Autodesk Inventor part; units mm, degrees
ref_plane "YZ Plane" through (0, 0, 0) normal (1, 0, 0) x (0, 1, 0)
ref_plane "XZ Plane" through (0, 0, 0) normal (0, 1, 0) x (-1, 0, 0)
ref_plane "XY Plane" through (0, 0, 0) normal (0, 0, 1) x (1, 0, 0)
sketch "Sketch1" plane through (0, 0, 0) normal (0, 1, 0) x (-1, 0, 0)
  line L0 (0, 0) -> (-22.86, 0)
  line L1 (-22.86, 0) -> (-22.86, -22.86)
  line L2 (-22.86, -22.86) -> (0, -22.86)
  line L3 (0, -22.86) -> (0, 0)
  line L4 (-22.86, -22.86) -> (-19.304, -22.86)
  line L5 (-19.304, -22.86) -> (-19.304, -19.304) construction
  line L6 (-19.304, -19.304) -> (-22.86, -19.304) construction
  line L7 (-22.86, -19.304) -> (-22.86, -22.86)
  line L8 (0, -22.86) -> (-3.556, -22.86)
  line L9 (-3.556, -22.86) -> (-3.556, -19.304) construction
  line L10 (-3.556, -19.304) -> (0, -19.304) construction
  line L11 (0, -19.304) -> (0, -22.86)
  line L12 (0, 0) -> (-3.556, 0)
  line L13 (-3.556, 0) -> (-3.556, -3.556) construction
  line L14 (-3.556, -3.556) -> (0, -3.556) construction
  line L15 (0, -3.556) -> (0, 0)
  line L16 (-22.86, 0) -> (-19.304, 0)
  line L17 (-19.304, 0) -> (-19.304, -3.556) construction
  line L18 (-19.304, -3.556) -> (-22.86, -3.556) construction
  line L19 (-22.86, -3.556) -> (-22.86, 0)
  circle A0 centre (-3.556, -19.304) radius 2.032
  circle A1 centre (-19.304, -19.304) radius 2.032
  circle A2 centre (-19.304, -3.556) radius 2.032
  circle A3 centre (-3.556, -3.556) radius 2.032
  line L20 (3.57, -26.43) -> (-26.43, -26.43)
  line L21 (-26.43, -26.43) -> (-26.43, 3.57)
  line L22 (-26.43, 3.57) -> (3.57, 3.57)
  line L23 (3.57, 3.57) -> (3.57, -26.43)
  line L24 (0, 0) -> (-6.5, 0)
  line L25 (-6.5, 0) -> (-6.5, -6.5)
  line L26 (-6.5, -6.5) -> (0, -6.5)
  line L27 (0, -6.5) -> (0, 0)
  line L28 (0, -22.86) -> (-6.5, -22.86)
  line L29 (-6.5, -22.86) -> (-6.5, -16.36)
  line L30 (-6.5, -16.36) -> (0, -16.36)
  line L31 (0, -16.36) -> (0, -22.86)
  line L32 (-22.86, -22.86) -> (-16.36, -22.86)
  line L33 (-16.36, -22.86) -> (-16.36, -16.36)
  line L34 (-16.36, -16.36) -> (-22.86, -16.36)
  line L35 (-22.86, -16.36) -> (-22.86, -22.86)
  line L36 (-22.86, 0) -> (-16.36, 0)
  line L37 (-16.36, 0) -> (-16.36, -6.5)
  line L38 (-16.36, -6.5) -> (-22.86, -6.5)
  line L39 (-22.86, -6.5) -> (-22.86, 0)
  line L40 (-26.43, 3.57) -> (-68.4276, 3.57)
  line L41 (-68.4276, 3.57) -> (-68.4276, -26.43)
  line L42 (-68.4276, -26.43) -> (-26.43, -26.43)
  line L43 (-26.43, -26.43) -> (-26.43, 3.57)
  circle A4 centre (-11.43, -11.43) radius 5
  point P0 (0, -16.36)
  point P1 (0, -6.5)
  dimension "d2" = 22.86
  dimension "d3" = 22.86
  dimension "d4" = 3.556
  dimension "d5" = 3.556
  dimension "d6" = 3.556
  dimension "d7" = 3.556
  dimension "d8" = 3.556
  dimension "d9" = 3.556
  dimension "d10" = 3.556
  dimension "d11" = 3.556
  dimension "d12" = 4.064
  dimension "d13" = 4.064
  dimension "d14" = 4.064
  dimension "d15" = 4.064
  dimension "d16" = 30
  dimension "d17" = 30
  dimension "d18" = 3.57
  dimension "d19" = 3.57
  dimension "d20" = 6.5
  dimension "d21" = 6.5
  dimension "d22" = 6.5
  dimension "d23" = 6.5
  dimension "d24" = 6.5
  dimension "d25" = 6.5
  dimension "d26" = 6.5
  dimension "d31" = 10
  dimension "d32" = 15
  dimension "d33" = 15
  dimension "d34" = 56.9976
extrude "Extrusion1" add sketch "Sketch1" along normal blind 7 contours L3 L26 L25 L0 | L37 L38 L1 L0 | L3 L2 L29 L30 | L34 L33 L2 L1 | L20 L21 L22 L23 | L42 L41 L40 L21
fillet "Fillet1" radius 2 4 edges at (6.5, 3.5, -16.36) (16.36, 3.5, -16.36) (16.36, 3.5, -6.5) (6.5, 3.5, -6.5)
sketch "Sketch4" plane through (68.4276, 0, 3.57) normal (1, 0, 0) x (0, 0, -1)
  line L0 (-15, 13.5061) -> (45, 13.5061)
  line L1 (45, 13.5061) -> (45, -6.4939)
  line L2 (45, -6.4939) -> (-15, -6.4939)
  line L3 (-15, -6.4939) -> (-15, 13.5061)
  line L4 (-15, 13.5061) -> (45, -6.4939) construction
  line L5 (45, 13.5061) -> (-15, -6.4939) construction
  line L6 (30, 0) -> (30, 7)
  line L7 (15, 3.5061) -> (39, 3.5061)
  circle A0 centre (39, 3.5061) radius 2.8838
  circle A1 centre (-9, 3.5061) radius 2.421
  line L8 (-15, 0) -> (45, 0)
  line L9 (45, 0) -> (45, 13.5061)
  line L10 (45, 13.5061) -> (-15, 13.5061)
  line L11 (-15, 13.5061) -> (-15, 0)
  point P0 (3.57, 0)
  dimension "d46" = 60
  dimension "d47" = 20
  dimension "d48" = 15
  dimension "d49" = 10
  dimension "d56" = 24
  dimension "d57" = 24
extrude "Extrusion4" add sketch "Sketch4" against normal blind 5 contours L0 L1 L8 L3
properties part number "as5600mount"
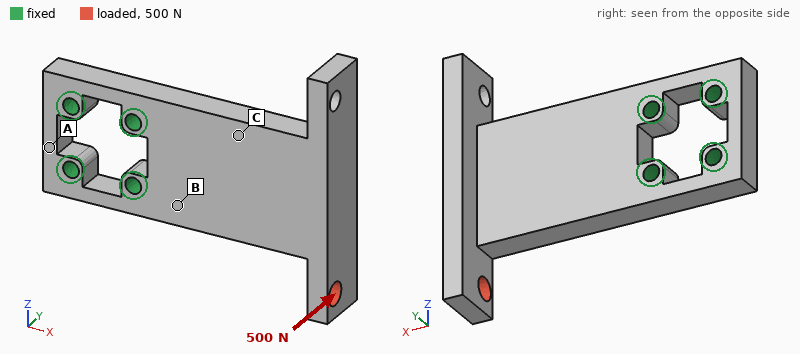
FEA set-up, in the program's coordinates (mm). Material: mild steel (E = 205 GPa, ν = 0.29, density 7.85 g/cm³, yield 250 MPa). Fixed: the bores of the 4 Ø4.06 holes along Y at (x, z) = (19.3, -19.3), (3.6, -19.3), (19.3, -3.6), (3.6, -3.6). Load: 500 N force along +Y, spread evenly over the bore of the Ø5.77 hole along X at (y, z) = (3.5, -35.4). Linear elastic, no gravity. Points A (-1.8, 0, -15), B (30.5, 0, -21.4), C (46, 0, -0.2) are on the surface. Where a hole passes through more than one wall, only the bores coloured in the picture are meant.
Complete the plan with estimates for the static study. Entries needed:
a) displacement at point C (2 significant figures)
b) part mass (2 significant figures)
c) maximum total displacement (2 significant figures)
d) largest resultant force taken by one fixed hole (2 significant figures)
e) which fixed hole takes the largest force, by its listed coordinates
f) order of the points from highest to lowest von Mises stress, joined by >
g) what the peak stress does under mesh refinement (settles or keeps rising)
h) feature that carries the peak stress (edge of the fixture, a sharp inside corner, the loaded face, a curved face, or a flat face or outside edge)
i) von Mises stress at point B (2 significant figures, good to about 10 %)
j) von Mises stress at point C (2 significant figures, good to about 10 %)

0.034 mm
120 g
0.19 mm
860 N
(19.3, -19.3)
B > C > A
keeps rising
edge of the fixture
92 MPa
52 MPa
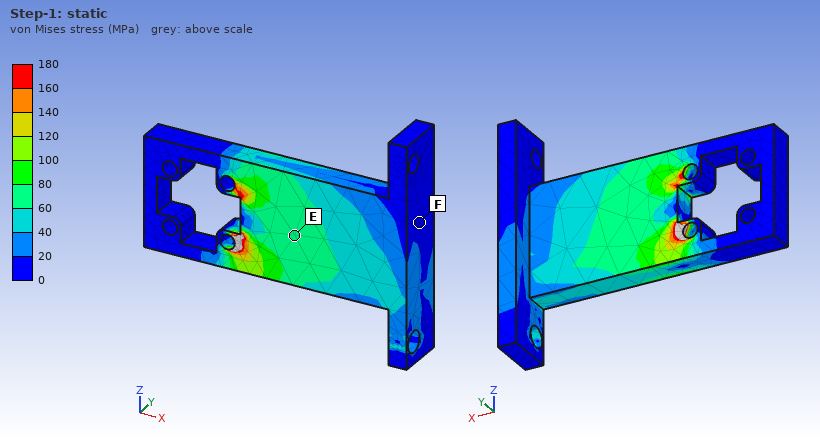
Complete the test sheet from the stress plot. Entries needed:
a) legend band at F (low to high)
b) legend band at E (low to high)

0 to 20 MPa
60 to 80 MPa
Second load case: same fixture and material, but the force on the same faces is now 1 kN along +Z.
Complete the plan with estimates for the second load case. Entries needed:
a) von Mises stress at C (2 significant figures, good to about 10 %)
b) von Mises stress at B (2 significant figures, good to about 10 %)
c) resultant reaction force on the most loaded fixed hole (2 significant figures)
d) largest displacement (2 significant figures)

15 MPa
24 MPa
2.0 kN
26 µm
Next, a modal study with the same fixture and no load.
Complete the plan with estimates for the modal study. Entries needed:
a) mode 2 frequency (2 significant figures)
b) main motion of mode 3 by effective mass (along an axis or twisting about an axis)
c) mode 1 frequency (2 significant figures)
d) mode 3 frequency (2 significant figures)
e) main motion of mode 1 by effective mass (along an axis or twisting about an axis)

3700 Hz
along Z
1600 Hz
5400 Hz
along Y
